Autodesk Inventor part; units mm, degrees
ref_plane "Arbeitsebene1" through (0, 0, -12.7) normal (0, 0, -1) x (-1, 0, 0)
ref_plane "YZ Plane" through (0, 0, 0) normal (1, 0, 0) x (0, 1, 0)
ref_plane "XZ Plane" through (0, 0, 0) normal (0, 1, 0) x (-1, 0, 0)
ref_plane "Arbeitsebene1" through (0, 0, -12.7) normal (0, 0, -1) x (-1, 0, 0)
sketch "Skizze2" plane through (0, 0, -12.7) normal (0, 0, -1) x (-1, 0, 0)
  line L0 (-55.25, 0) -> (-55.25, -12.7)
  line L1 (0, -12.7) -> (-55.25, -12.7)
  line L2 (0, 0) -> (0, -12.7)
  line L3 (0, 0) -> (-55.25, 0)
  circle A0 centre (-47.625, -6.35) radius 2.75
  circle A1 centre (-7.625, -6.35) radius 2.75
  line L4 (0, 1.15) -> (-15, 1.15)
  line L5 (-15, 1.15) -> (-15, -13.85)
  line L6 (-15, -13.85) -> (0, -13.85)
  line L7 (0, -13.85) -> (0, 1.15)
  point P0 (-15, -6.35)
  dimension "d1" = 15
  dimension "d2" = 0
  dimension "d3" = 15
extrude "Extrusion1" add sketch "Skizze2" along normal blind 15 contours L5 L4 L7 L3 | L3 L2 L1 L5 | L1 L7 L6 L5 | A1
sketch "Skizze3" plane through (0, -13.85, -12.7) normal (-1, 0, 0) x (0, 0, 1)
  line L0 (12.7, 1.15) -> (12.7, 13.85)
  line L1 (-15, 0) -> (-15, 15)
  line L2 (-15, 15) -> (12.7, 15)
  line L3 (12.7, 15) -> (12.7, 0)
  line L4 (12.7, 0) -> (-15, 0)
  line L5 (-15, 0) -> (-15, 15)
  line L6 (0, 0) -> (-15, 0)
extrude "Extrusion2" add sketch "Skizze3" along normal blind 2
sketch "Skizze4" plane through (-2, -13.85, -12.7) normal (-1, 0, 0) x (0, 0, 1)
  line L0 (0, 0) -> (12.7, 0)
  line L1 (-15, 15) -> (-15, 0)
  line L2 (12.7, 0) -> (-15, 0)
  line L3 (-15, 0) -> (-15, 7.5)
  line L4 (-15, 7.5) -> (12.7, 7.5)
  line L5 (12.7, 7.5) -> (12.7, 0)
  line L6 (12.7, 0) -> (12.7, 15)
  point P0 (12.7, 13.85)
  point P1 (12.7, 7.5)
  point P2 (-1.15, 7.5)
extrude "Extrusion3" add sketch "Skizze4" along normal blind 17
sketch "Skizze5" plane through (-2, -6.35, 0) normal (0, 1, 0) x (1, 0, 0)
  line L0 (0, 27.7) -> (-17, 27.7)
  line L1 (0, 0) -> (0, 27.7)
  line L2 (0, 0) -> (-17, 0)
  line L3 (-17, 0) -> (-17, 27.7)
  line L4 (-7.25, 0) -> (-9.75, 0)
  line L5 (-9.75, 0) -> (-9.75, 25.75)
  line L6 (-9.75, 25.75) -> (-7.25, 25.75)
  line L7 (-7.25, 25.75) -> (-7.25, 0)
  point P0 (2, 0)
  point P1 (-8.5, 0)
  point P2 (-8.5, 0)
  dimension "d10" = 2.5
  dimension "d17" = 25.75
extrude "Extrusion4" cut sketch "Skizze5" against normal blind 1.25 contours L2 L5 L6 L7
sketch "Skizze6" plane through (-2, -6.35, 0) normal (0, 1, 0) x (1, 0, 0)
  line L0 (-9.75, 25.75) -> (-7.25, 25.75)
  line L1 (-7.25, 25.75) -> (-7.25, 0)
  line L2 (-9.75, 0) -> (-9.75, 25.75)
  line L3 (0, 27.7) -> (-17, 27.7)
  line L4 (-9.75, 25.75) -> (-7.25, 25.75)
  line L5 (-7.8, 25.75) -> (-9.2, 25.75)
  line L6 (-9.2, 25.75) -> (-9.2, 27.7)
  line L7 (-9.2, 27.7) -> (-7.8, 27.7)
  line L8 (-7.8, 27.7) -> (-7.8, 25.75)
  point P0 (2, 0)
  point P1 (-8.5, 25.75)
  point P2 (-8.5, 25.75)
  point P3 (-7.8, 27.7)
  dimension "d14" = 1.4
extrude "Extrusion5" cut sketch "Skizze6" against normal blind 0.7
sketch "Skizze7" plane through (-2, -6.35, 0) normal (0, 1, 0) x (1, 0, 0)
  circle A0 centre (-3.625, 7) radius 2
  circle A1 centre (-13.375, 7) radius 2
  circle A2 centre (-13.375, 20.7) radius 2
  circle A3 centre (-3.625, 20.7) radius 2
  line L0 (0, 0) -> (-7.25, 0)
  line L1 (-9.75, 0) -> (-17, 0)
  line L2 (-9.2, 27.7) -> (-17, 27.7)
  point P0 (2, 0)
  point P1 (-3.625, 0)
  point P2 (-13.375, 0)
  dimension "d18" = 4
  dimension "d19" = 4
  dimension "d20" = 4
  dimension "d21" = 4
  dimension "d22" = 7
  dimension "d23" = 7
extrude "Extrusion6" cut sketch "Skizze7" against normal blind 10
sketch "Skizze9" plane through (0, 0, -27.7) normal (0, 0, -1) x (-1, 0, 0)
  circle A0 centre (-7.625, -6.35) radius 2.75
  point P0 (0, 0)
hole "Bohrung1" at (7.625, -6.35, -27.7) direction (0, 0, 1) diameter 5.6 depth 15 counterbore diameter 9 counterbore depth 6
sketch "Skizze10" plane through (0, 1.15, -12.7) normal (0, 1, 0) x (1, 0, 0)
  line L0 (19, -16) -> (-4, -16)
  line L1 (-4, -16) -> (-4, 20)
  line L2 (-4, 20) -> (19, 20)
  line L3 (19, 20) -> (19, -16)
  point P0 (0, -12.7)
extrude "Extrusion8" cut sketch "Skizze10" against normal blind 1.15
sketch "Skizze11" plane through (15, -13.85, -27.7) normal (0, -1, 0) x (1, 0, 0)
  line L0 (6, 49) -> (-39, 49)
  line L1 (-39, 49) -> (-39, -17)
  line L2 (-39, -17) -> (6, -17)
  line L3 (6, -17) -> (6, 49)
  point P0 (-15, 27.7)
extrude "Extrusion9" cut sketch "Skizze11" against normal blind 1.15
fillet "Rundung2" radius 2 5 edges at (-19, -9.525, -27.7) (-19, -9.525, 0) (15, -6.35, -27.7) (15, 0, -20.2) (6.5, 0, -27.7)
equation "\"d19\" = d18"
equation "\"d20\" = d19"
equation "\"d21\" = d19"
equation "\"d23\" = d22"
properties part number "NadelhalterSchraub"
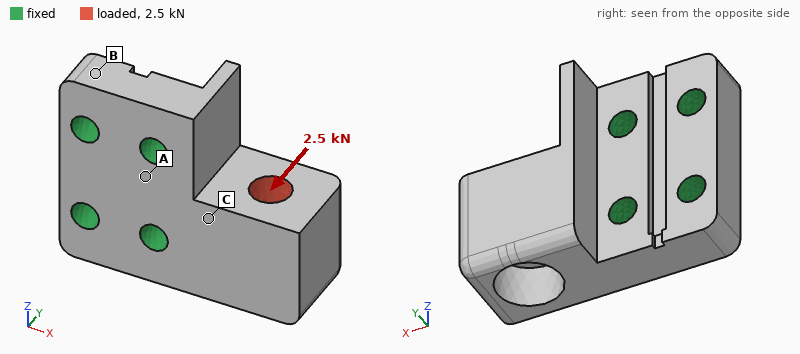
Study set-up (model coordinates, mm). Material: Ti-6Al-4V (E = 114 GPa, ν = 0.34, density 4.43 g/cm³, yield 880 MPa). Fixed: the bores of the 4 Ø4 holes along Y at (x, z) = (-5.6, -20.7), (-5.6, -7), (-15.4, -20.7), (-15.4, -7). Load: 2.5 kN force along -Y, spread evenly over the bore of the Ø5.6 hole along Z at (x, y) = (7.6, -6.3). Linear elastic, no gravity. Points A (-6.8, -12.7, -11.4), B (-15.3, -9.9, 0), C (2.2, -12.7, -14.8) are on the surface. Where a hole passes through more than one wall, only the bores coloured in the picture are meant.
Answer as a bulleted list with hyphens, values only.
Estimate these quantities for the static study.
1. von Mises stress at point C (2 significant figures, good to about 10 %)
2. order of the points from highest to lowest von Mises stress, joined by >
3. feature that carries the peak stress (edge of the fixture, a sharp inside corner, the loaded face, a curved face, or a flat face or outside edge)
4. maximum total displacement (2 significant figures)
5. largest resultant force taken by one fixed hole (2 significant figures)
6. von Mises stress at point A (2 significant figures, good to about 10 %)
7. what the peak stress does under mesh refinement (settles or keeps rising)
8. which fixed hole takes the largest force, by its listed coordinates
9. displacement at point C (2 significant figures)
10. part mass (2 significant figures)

- 99 MPa
- C > A > B
- edge of the fixture
- 87 µm
- 2.3 kN
- 64 MPa
- keeps rising
- (-5.6, -20.7)
- 25 µm
- 24 g
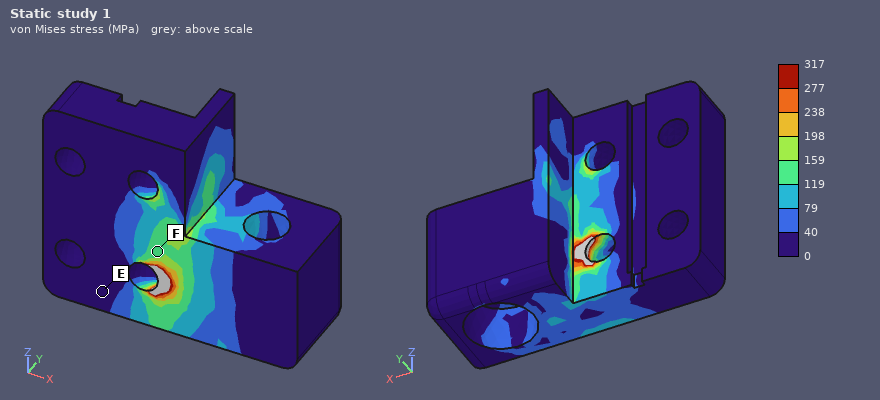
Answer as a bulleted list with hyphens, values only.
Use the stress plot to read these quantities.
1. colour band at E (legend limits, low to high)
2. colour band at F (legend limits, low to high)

- 0 to 40 MPa
- 119 to 159 MPa
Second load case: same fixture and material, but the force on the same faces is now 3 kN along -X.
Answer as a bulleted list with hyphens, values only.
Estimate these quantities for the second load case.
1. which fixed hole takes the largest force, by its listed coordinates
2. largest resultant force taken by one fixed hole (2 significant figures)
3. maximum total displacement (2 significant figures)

- (-5.6, -20.7)
- 2.0 kN
- 30 µm
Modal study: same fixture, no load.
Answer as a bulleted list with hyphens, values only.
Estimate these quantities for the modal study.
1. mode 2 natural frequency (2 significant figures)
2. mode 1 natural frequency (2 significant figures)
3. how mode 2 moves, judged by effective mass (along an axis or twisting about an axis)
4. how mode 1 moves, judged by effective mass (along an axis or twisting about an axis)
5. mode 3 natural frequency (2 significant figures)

- 18 kHz
- 9800 Hz
- along Z
- along Y
- 28 kHz
